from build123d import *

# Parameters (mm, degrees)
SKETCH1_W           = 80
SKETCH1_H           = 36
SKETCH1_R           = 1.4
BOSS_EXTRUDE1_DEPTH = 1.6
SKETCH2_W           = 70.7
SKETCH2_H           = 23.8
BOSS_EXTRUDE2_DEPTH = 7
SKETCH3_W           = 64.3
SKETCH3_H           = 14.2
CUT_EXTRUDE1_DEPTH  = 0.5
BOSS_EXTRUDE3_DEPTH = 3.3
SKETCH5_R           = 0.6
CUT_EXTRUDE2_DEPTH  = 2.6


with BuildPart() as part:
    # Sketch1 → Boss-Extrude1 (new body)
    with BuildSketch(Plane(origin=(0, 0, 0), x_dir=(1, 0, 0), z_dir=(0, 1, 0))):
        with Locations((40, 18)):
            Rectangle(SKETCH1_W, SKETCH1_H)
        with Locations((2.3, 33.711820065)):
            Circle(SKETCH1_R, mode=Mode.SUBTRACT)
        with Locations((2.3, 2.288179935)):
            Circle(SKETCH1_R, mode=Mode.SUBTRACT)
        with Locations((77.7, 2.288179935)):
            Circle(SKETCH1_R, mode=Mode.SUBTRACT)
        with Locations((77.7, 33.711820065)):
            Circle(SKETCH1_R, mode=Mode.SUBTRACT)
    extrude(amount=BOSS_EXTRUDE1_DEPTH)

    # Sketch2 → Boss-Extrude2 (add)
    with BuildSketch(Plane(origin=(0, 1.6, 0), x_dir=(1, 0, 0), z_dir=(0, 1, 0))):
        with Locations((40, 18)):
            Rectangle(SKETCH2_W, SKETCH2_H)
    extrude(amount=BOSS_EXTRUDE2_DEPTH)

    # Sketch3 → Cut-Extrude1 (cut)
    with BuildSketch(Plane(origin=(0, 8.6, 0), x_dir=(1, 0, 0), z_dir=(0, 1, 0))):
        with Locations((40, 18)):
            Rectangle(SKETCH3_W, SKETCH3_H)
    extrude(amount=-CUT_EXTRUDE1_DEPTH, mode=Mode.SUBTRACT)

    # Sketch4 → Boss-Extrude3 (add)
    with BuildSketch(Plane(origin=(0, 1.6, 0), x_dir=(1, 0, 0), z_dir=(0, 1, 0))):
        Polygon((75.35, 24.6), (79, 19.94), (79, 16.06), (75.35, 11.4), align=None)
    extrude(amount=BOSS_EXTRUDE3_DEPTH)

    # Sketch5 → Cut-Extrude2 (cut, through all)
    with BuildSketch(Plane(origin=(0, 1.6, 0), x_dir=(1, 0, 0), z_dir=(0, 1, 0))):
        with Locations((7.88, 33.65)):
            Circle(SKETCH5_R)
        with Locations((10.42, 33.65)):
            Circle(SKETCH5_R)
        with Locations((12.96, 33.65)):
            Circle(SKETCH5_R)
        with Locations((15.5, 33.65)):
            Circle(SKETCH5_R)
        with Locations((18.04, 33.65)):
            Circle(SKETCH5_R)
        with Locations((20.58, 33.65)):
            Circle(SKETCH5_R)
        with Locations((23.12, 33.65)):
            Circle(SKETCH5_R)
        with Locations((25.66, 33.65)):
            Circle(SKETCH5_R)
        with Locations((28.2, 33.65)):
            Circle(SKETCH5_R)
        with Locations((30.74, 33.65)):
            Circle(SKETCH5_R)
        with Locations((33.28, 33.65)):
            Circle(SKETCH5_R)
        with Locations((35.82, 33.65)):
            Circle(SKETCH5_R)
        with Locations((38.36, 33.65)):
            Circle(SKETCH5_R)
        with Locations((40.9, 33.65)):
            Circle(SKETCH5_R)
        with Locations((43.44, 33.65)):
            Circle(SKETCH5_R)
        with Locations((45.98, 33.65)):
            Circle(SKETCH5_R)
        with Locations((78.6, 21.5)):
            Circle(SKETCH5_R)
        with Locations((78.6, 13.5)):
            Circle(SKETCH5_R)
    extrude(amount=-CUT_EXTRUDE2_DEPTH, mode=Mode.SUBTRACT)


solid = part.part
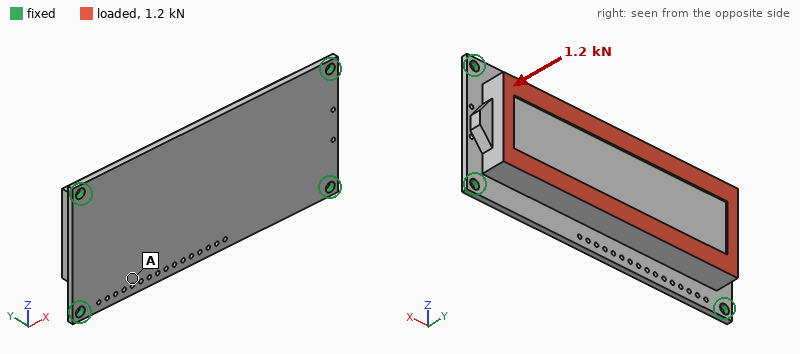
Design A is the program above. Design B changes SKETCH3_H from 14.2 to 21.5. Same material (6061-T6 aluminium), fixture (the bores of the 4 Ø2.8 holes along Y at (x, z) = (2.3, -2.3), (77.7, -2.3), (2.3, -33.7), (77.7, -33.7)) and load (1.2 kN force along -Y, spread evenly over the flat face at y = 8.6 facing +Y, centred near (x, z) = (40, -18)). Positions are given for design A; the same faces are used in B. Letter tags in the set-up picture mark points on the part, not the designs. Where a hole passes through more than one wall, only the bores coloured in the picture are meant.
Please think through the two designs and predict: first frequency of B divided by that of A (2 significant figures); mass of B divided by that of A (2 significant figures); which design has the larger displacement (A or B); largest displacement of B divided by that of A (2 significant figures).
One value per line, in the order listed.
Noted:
0.99
0.99
A
0.81
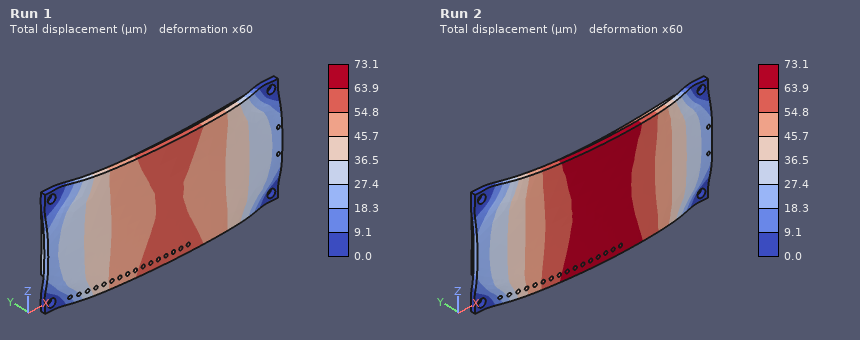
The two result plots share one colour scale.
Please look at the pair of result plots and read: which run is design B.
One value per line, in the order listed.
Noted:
Run 1
